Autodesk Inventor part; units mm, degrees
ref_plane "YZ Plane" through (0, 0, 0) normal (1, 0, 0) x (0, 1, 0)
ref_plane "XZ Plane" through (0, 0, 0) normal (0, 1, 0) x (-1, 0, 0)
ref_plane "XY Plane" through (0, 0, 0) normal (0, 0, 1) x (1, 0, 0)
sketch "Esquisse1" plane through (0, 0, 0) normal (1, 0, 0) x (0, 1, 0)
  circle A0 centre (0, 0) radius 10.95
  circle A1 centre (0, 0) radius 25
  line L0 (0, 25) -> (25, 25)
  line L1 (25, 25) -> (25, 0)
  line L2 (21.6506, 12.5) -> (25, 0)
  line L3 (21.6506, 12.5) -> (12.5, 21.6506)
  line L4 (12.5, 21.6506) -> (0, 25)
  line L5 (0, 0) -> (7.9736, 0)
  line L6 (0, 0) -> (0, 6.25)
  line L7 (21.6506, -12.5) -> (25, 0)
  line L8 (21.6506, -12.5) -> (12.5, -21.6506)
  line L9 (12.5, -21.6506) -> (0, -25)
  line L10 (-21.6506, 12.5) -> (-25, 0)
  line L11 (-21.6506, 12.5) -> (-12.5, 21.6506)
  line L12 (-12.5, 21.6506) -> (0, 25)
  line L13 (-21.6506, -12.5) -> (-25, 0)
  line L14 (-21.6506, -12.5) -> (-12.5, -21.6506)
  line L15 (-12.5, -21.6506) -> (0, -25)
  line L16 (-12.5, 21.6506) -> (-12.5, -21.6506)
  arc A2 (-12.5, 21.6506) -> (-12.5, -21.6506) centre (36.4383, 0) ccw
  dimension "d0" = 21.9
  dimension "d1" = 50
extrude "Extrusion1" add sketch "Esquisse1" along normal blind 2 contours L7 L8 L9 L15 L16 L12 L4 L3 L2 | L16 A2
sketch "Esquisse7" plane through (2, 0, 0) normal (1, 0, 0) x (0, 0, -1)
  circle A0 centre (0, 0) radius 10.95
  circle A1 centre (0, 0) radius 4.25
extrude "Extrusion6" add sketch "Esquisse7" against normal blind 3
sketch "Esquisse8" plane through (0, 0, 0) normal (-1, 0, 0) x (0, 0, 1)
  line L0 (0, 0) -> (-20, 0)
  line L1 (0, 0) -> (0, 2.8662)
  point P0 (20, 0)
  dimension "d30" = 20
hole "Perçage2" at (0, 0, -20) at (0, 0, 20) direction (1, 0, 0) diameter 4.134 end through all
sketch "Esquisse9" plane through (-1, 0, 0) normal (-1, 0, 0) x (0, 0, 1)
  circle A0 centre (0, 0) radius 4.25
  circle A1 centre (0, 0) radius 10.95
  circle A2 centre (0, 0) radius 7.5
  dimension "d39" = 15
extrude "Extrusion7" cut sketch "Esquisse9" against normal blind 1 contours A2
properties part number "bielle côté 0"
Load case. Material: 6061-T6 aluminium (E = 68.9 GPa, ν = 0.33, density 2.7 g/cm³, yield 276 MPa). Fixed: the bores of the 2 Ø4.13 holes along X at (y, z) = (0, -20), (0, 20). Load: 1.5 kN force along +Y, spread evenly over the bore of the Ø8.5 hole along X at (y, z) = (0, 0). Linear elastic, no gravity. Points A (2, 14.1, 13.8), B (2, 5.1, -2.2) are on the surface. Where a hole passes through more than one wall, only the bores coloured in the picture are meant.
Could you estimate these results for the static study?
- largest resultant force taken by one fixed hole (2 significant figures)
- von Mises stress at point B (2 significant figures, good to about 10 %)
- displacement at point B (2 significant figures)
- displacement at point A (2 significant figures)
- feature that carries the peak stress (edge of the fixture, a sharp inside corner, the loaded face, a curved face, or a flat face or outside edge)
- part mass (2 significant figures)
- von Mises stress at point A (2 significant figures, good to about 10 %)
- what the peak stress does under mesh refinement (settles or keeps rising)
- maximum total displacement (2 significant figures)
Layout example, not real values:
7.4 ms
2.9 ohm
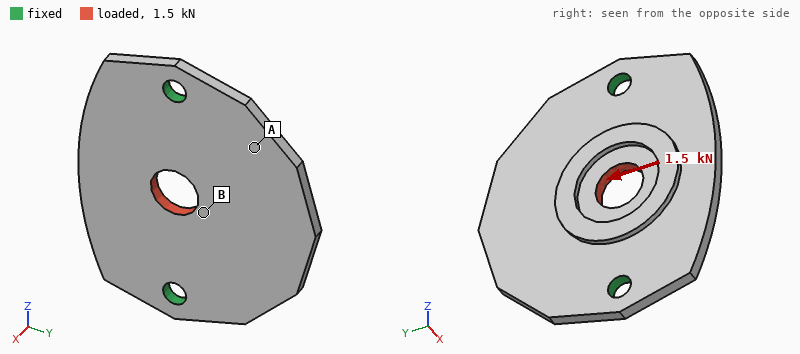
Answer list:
750 N
29 MPa
11 µm
5.7 µm
edge of the fixture
9.0 g
15 MPa
keeps rising
13 µm
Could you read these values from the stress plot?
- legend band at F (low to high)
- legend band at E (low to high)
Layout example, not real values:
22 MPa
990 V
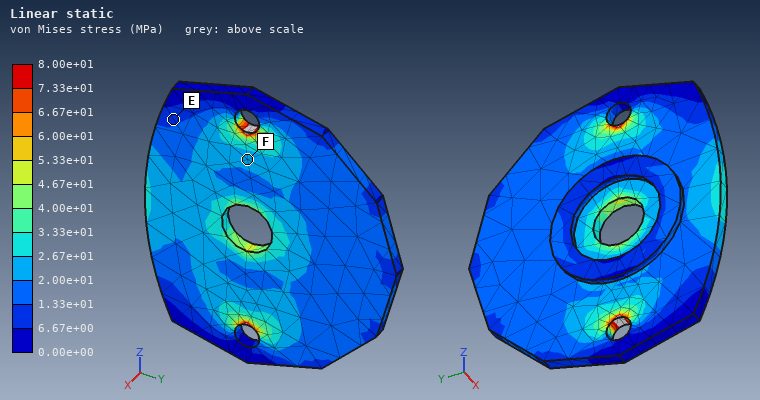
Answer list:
2.00e+01 to 2.67e+01 MPa
6.67e+00 to 1.33e+01 MPa
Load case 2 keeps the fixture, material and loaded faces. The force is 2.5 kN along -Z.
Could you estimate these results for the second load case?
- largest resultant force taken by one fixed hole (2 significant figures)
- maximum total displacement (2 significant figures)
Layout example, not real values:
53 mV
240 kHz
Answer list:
1.3 kN
13 µm
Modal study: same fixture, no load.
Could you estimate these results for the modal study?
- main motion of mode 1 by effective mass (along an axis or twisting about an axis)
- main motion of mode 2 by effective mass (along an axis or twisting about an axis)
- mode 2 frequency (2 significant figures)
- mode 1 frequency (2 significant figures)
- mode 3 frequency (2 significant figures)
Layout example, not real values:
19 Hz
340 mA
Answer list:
along X
along X
5000 Hz
2900 Hz
7900 Hz
